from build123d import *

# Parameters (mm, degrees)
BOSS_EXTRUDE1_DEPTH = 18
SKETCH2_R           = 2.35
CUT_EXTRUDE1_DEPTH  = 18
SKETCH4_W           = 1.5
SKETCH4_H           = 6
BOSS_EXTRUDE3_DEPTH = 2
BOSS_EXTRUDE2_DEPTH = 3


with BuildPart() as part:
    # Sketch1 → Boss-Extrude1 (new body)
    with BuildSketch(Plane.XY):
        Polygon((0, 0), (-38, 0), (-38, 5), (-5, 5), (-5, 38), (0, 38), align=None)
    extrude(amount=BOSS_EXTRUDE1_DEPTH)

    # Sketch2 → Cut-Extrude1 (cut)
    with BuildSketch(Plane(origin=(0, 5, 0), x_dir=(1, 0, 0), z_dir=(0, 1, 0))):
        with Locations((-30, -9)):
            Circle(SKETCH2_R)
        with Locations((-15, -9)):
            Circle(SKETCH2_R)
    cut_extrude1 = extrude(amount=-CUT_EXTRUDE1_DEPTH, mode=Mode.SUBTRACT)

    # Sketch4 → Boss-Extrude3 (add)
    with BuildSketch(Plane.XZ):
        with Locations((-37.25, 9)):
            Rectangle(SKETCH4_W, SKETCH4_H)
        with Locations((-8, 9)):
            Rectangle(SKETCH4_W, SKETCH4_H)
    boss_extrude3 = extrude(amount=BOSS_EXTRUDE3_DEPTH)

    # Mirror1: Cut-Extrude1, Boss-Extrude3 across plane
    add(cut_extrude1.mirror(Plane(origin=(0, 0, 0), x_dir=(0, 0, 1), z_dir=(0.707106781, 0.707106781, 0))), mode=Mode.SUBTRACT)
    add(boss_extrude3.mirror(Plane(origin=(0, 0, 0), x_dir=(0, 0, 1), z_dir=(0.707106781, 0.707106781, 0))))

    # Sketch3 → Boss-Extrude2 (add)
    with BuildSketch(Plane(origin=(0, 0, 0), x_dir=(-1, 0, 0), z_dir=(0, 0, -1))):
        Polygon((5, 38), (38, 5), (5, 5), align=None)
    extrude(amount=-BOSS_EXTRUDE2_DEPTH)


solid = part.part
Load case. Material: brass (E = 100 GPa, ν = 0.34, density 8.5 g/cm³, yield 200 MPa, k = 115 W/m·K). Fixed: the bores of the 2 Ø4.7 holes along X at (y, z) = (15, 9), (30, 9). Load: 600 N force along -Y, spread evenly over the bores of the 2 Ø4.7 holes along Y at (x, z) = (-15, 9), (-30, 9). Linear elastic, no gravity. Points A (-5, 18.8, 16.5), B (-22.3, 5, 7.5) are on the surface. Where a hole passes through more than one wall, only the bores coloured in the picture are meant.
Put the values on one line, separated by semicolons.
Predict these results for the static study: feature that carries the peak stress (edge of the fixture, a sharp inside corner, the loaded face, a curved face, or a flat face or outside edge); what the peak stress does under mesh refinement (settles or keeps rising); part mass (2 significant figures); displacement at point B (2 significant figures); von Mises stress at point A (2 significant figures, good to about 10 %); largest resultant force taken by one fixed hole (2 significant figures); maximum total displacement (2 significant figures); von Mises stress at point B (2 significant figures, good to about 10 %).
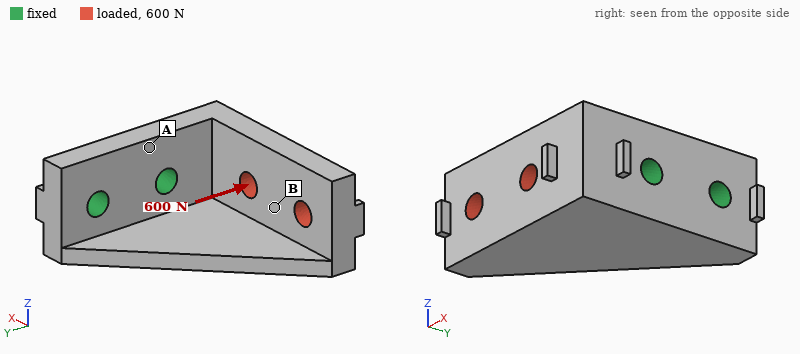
edge of the fixture; keeps rising; 66 g; 31 µm; 10 MPa; 610 N; 84 µm; 27 MPa
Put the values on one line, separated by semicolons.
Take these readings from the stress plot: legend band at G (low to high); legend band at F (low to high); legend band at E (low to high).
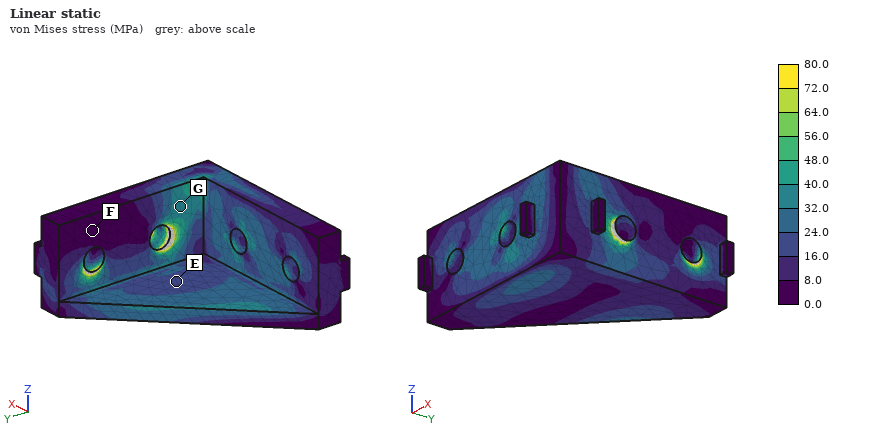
32.0 to 40.0 MPa; 0.0 to 8.0 MPa; 16.0 to 24.0 MPa
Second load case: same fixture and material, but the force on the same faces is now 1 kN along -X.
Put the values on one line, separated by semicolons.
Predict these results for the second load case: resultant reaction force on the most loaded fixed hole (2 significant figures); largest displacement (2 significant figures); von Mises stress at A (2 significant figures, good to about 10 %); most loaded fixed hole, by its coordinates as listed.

1.4 kN; 42 µm; 20 MPa; (15, 9)
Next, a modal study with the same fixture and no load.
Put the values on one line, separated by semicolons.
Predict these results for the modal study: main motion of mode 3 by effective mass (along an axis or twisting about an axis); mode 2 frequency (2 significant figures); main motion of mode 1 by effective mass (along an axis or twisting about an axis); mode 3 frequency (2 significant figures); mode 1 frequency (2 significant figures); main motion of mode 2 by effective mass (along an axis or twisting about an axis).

along X; 3700 Hz; along Z; 7100 Hz; 2400 Hz; along Y
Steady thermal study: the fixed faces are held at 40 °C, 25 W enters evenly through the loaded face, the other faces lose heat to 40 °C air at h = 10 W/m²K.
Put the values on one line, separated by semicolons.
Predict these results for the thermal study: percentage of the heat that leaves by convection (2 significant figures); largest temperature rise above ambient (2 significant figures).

3.7 %; 51 K
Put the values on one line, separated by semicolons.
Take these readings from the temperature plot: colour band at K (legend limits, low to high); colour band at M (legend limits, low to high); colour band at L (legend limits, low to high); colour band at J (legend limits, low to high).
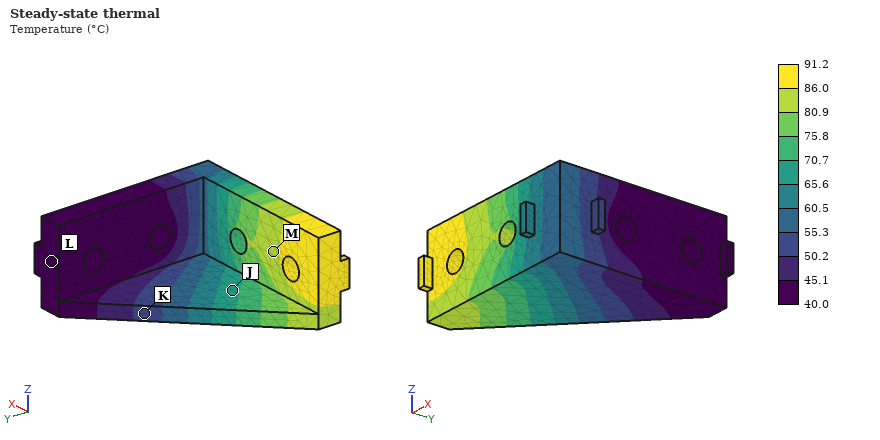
50.2 to 55.3 °C; 80.9 to 86.0 °C; 40.0 to 45.1 °C; 65.6 to 70.7 °C
